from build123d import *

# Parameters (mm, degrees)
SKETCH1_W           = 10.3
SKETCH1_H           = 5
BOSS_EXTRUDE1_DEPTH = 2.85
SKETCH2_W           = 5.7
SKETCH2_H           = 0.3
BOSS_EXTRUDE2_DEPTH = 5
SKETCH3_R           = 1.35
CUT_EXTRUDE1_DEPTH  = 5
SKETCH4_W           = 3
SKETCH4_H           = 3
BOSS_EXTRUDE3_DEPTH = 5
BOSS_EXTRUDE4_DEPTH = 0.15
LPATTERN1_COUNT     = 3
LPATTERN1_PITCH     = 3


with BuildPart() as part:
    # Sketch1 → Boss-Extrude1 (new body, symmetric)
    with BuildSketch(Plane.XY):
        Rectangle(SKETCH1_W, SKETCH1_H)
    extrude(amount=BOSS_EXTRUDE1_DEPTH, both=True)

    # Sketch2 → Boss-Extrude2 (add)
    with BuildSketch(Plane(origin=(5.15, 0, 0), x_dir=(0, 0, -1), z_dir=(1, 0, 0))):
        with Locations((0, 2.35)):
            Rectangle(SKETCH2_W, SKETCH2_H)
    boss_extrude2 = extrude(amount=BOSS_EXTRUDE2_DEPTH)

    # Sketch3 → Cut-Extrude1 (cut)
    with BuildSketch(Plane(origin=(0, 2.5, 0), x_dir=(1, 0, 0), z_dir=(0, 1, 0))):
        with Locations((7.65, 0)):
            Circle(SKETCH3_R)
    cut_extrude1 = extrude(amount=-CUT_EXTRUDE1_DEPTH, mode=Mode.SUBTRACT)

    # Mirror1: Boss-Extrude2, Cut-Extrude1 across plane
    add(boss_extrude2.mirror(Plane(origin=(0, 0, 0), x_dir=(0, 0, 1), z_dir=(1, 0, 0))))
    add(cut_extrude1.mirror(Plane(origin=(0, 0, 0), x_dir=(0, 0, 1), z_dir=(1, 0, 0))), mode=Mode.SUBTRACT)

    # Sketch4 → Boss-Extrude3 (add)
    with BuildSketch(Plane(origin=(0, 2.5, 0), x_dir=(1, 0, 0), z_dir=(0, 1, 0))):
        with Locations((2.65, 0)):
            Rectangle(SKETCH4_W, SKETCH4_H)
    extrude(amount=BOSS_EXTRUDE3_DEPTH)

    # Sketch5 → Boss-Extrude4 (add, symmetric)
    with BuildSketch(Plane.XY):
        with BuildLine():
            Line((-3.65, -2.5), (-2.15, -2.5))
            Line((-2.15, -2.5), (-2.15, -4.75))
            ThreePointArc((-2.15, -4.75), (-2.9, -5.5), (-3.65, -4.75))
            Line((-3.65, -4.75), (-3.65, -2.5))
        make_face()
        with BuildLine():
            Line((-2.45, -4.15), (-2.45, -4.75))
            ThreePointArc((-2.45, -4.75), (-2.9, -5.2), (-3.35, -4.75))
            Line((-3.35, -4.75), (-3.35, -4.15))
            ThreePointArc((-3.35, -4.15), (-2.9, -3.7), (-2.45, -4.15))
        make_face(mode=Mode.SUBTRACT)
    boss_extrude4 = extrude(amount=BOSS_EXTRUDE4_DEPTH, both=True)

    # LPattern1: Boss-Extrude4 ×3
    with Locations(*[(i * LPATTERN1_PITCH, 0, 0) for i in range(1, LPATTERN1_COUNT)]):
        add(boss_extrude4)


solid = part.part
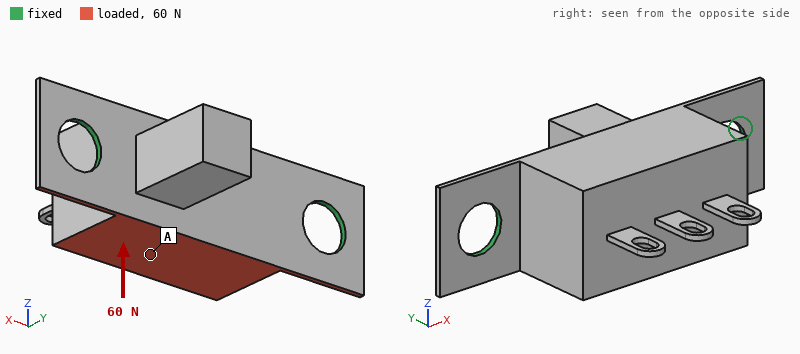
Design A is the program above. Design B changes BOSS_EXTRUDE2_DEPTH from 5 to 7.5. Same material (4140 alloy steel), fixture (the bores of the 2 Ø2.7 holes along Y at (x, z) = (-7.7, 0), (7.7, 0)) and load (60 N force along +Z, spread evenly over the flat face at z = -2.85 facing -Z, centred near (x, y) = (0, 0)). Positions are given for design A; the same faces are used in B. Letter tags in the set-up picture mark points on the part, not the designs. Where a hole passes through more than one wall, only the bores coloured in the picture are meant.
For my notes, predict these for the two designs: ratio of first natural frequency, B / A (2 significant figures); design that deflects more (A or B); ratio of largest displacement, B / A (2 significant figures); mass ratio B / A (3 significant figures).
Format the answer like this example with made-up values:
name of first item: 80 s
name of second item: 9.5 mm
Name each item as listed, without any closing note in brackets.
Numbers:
ratio of first natural frequency, B / A: 1.0
design that deflects more: A
ratio of largest displacement, B / A: 0.91
mass ratio B / A: 1.02
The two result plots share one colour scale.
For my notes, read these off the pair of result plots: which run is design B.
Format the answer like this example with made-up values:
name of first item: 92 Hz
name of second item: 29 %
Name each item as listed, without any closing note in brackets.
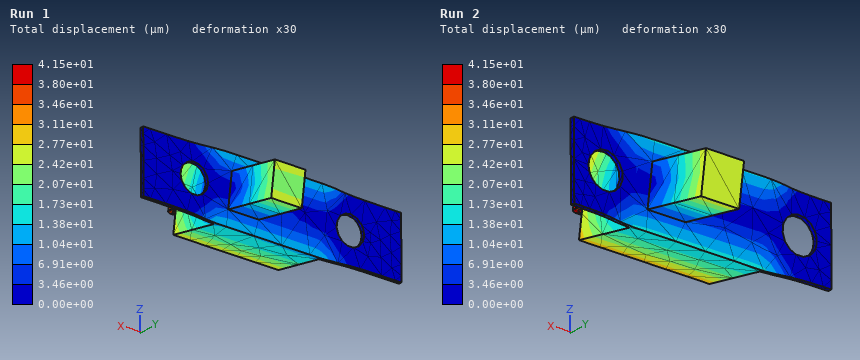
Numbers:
which run is design B: Run 1
